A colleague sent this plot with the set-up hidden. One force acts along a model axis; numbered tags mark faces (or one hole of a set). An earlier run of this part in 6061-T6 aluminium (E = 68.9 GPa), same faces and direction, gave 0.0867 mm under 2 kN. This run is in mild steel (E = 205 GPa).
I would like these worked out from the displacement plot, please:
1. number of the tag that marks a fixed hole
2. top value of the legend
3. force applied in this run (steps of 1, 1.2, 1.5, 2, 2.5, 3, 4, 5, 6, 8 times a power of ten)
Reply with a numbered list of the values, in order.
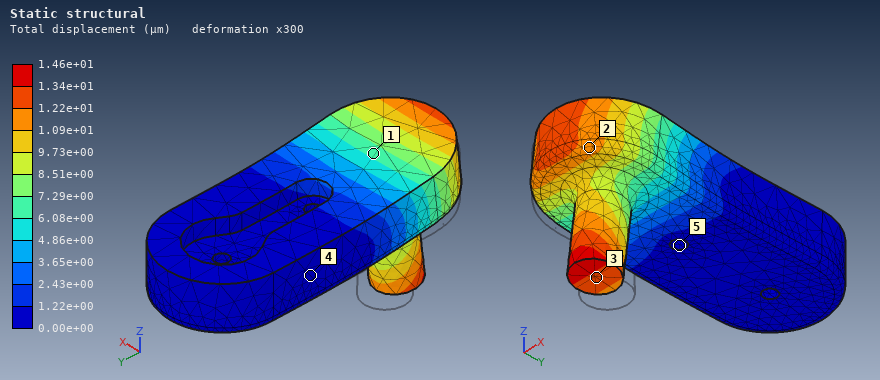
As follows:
1. 5
2. 1.46e+01 µm
3. 1 kN
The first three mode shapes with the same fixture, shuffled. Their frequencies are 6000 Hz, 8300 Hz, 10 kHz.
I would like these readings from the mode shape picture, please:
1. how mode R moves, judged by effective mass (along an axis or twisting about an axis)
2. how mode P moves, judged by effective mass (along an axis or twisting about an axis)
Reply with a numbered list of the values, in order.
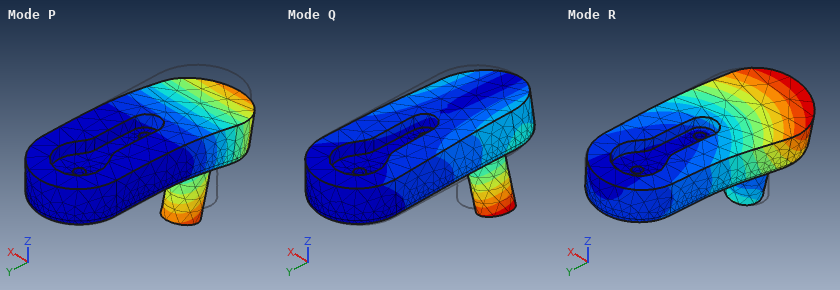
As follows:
1. along X
2. along Z
